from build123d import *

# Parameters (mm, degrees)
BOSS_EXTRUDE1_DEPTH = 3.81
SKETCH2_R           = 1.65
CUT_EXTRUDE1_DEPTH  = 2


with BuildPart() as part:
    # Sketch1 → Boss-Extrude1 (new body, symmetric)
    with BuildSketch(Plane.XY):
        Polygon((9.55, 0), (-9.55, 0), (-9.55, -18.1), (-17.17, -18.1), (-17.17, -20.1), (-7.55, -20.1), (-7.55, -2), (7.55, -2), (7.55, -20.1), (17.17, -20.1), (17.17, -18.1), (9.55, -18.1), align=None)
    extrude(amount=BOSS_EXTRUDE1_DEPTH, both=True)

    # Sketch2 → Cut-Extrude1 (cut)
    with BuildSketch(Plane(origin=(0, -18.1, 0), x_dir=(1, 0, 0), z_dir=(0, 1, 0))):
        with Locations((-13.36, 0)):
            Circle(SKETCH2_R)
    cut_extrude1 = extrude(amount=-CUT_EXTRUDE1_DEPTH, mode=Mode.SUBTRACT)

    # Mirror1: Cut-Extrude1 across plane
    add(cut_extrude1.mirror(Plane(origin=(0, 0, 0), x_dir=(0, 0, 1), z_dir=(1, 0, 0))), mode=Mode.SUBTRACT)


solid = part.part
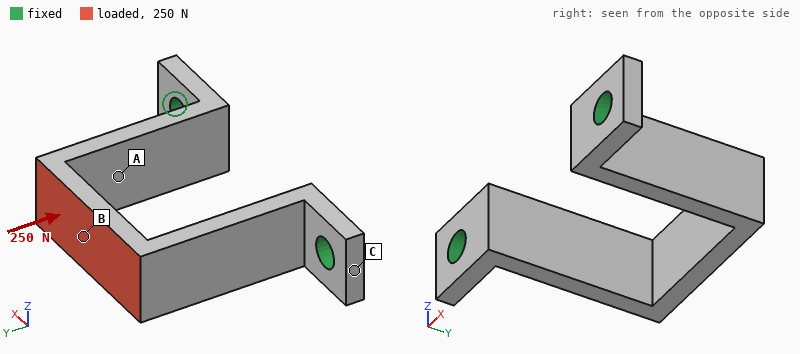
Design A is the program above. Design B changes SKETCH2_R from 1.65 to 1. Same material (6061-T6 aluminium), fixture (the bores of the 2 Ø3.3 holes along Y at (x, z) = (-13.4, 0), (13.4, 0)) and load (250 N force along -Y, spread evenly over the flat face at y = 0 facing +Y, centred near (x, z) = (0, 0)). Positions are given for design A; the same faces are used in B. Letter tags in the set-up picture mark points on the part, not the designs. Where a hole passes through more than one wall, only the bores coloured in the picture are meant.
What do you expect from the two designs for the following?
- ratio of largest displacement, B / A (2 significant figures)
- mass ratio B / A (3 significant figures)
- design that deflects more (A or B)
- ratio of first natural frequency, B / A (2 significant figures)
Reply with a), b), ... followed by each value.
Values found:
a) 1.1
b) 1.02
c) B
d) 0.91
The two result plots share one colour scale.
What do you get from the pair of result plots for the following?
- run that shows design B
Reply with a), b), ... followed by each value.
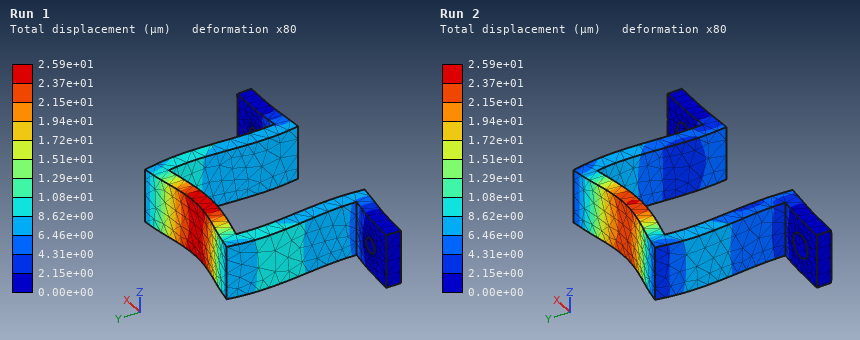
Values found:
a) Run 1
